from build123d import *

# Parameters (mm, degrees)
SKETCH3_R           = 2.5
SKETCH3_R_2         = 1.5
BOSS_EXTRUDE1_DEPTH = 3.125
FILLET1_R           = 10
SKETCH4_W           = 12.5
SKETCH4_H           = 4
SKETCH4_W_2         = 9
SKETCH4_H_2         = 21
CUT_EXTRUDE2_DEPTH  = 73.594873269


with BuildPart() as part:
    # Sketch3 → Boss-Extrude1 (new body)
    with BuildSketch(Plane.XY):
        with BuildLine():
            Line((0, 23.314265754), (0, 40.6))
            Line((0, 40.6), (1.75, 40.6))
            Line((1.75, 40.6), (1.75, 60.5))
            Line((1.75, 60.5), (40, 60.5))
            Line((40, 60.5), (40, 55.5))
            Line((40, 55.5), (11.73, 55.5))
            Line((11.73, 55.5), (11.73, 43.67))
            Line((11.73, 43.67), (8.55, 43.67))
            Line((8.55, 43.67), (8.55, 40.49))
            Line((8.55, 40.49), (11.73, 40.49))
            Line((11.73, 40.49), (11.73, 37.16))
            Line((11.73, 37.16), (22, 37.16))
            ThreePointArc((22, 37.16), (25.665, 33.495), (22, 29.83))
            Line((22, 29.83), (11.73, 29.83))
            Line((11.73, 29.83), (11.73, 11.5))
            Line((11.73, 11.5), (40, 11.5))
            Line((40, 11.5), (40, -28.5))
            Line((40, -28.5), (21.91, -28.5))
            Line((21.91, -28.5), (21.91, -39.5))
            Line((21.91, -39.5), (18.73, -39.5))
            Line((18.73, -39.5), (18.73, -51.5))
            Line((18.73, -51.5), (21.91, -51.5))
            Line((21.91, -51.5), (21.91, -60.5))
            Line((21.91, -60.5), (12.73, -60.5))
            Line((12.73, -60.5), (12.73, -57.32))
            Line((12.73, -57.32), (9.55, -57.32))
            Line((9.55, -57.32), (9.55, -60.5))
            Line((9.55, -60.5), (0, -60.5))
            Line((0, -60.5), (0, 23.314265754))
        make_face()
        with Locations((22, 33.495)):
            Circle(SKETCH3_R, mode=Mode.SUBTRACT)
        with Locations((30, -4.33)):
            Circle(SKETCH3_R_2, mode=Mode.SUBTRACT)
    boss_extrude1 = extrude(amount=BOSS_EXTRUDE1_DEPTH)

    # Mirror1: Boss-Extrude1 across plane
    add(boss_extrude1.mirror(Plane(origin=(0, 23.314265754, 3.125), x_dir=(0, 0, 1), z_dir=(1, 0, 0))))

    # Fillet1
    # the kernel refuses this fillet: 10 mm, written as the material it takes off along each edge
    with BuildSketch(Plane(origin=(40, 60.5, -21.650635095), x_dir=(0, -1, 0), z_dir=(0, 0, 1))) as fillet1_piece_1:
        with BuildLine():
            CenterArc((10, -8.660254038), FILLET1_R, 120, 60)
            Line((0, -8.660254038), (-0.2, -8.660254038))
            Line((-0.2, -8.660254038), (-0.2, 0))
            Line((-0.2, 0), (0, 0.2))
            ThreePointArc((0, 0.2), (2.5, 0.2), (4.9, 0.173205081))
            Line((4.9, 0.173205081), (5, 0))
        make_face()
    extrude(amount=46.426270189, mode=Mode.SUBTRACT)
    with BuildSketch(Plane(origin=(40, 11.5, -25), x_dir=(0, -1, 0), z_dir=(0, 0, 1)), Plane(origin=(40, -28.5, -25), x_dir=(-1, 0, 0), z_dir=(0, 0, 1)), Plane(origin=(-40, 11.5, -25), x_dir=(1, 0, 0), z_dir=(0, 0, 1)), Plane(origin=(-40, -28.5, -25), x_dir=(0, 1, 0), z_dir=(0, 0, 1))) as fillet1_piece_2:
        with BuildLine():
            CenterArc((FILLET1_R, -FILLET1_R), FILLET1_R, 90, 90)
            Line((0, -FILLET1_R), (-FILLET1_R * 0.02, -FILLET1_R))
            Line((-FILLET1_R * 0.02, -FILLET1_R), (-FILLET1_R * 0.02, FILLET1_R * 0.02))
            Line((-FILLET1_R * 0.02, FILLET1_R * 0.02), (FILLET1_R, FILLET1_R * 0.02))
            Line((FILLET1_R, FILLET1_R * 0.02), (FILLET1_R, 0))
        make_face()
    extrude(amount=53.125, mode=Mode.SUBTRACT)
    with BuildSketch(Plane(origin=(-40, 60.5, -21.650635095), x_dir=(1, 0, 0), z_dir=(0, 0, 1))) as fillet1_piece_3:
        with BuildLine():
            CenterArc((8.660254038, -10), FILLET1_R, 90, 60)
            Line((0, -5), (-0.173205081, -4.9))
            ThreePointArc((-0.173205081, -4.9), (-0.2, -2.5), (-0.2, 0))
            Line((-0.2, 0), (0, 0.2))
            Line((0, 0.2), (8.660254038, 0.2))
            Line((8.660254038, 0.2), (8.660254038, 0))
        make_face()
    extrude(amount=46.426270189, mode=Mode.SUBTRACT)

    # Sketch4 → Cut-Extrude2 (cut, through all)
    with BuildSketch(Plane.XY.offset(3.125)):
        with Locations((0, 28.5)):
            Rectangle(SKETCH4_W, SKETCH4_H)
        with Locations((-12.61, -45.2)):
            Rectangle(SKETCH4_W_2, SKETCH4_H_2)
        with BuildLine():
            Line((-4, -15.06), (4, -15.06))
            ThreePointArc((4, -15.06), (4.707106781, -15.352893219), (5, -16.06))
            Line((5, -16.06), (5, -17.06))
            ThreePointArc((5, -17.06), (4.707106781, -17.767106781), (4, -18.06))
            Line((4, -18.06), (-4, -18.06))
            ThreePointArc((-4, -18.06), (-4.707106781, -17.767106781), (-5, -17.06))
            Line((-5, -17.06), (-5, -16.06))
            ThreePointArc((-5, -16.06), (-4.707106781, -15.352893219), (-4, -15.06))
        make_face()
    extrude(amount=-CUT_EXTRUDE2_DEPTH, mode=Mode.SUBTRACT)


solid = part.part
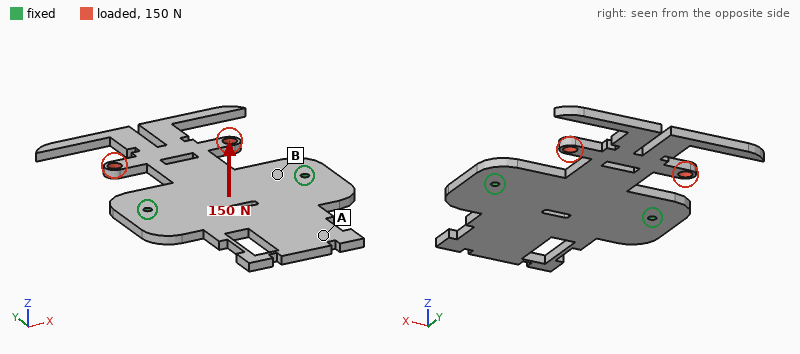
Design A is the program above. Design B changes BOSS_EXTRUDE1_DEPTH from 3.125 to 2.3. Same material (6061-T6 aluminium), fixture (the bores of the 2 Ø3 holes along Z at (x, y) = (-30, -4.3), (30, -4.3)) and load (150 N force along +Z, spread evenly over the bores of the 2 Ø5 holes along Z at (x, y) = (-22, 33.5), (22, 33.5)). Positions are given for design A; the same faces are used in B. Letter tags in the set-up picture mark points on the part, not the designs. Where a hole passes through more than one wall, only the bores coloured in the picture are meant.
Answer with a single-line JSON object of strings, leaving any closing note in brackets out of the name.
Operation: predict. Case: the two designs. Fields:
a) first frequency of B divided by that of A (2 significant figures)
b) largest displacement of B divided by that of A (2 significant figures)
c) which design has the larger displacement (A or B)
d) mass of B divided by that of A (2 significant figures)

{"first frequency of B divided by that of A": "0.75", "largest displacement of B divided by that of A": "2.4", "which design has the larger displacement": "B", "mass of B divided by that of A": "0.74"}
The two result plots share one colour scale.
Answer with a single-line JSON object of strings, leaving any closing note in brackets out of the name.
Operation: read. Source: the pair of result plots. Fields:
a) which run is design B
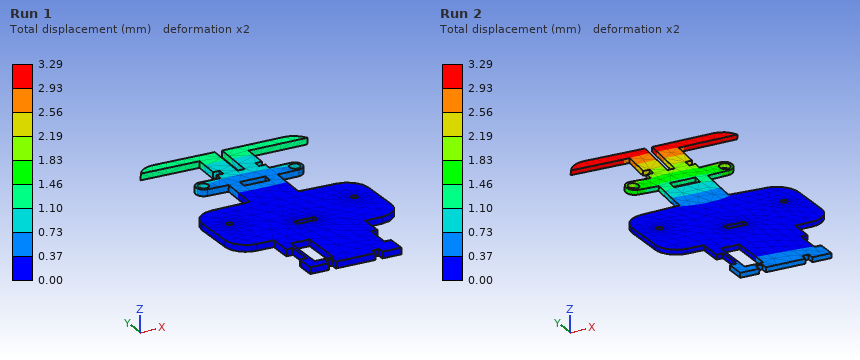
{"which run is design B": "Run 2"}
